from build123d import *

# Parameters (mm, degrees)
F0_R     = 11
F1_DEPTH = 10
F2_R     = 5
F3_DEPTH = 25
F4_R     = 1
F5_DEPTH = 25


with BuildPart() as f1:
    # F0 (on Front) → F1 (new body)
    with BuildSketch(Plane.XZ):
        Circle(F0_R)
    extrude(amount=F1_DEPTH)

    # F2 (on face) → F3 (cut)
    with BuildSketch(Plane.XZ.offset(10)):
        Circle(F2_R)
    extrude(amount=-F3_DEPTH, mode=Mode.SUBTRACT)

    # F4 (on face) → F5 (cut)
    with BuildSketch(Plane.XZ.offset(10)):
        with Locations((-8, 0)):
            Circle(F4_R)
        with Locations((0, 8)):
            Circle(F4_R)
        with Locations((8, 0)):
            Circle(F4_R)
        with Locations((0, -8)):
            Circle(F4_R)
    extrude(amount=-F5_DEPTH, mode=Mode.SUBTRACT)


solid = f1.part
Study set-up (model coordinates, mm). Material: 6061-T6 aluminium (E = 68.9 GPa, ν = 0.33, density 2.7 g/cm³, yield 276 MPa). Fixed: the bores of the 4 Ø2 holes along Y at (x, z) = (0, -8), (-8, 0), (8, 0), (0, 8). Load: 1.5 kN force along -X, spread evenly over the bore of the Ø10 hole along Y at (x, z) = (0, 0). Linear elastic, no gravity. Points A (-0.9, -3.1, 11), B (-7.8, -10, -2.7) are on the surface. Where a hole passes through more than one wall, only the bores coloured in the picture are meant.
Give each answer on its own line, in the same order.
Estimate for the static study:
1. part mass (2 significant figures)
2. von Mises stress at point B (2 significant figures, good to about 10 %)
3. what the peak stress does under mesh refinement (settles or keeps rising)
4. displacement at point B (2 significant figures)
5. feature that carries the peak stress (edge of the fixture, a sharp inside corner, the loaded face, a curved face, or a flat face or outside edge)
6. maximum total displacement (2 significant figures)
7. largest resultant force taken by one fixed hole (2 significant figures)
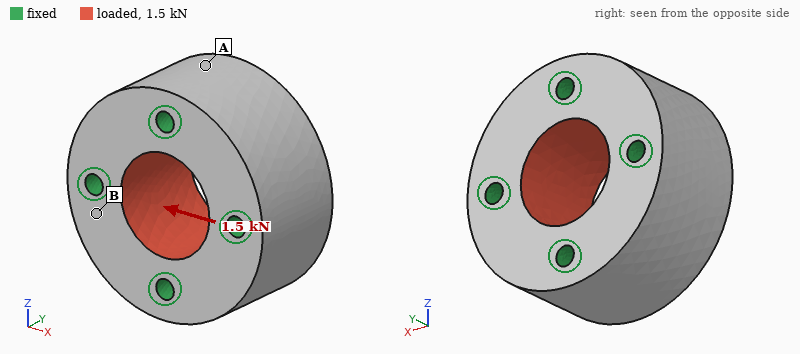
7.8 g
4.8 MPa
keeps rising
0.27 µm
edge of the fixture
0.62 µm
380 N
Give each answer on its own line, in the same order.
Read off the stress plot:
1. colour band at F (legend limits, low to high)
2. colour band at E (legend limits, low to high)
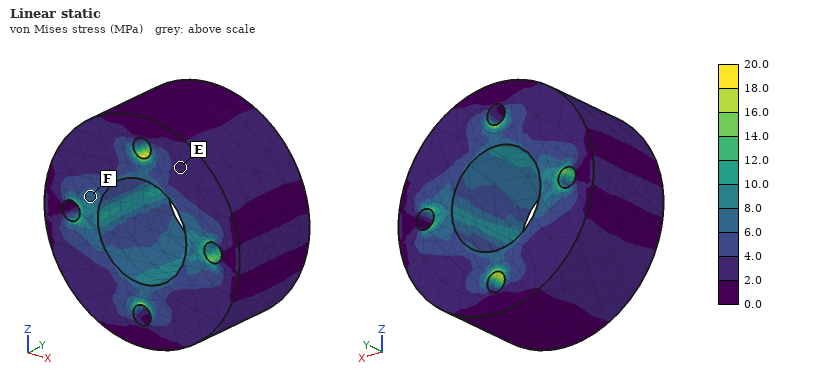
6.0 to 8.0 MPa
2.0 to 4.0 MPa
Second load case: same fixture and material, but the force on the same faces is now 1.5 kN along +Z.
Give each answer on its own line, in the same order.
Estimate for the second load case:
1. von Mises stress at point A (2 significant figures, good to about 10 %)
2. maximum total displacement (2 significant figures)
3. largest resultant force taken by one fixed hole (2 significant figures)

2.6 MPa
0.62 µm
380 N
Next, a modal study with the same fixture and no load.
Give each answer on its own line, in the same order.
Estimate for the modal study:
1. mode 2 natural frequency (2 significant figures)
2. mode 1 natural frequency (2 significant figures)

100 kHz
98 kHz
